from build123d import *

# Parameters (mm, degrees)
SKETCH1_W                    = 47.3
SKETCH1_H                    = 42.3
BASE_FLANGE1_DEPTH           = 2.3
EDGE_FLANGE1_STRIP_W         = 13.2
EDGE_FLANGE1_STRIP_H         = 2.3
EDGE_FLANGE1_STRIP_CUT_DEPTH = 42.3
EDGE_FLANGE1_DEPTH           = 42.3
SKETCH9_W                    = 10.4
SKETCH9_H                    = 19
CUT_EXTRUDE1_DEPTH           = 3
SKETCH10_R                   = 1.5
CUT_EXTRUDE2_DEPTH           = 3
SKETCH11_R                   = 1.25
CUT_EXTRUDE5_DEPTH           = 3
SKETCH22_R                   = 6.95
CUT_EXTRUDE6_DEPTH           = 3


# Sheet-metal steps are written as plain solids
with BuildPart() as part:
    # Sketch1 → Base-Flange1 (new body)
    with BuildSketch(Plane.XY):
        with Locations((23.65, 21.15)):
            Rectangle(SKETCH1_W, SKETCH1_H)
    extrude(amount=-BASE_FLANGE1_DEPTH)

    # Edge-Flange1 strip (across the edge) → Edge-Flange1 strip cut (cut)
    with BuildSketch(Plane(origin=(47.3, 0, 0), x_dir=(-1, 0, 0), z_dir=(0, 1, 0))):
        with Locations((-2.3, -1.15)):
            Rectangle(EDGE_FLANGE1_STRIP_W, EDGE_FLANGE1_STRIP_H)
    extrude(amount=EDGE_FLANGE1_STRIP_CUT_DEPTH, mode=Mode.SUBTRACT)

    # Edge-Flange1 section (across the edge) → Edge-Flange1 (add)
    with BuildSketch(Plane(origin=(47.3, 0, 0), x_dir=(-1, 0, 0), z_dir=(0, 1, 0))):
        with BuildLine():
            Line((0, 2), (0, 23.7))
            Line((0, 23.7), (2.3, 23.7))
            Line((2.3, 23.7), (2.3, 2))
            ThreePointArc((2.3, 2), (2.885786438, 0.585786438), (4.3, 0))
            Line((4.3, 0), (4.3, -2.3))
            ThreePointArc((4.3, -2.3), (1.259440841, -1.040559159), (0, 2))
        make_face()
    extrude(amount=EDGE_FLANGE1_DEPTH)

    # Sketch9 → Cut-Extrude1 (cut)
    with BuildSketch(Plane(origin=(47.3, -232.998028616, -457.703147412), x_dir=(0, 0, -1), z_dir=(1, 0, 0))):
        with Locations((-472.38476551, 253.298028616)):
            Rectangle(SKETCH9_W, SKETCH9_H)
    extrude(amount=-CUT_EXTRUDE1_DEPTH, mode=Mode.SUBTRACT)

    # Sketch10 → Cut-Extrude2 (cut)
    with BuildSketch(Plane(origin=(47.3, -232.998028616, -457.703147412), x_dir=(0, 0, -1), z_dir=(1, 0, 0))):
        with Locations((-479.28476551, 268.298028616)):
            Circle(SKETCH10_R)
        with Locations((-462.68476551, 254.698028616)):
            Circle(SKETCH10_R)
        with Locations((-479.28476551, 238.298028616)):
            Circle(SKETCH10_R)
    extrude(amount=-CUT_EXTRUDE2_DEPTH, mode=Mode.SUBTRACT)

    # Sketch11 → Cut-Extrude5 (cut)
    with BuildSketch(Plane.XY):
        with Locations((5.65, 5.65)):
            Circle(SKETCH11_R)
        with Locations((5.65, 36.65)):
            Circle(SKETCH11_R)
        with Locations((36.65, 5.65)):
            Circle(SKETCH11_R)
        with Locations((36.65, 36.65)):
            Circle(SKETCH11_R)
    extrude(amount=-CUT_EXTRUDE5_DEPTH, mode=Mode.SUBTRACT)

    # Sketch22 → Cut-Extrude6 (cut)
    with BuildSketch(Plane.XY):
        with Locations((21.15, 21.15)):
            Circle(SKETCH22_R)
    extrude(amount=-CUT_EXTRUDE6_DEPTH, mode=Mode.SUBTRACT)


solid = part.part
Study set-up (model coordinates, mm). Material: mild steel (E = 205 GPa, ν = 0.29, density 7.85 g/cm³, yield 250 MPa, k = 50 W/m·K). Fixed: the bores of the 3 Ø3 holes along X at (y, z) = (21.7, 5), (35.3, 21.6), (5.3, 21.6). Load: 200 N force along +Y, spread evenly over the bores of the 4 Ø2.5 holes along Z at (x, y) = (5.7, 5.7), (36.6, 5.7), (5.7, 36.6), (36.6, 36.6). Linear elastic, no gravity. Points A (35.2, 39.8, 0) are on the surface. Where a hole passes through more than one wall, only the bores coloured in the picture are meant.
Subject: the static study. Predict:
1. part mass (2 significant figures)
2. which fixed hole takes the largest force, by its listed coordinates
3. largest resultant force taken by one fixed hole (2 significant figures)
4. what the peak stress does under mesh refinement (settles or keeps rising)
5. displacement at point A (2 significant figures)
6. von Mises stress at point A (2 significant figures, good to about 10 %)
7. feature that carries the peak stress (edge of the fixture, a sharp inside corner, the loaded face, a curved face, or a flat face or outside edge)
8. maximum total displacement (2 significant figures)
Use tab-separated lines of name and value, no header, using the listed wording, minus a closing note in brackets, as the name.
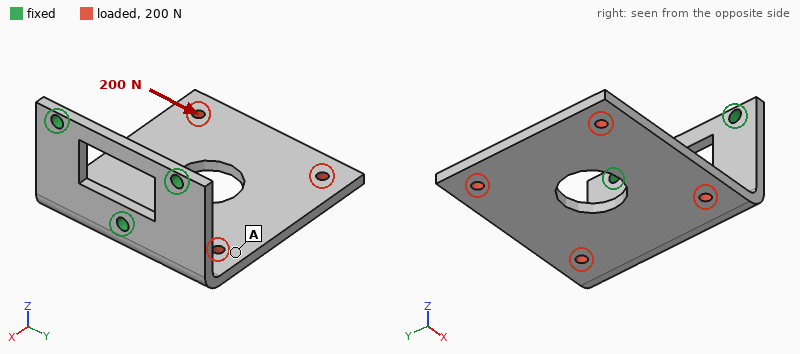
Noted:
part mass	46 g
which fixed hole takes the largest force, by its listed coordinates	(21.7, 5)
largest resultant force taken by one fixed hole	170 N
what the peak stress does under mesh refinement	keeps rising
displacement at point A	0.054 mm
von Mises stress at point A	29 MPa
feature that carries the peak stress	edge of the fixture
maximum total displacement	0.13 mm
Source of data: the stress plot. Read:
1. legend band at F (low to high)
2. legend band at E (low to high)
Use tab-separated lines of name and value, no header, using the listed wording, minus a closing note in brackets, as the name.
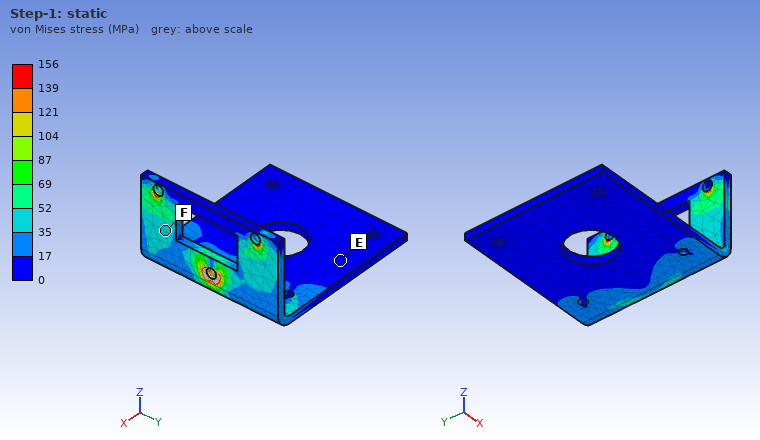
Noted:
legend band at F	35 to 52 MPa
legend band at E	0 to 17 MPa
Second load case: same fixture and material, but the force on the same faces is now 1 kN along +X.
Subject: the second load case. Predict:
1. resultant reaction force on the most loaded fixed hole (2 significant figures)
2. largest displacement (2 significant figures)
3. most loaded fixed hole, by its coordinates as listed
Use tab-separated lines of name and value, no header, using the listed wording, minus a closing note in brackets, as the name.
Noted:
resultant reaction force on the most loaded fixed hole	1.1 kN
largest displacement	0.16 mm
most loaded fixed hole, by its coordinates as listed	(21.7, 5)
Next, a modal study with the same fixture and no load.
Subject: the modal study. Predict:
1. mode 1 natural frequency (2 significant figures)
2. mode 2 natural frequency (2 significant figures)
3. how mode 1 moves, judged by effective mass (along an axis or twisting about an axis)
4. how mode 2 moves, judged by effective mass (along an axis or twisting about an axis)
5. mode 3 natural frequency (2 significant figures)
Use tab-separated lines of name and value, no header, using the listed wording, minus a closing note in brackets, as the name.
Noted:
mode 1 natural frequency	730 Hz
mode 2 natural frequency	1300 Hz
how mode 1 moves, judged by effective mass	along Z
how mode 2 moves, judged by effective mass	along Y
mode 3 natural frequency	2100 Hz
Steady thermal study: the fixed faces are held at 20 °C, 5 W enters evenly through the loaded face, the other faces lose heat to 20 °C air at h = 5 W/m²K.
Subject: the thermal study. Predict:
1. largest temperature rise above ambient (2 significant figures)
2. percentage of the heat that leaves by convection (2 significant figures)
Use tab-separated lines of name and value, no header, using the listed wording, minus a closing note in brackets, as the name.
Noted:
largest temperature rise above ambient	41 K
percentage of the heat that leaves by convection	12 %
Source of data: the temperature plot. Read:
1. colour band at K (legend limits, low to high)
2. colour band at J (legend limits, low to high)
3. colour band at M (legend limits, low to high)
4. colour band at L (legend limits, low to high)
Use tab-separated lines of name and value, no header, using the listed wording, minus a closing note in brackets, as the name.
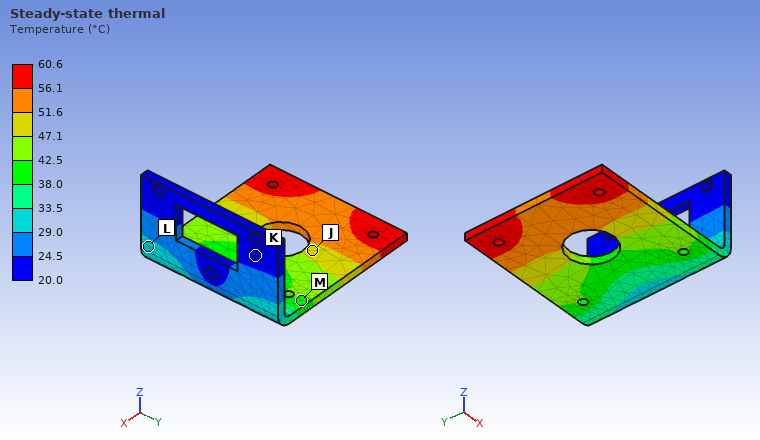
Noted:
colour band at K	20.0 to 24.5 °C
colour band at J	47.1 to 51.6 °C
colour band at M	38.0 to 42.5 °C
colour band at L	29.0 to 33.5 °C
